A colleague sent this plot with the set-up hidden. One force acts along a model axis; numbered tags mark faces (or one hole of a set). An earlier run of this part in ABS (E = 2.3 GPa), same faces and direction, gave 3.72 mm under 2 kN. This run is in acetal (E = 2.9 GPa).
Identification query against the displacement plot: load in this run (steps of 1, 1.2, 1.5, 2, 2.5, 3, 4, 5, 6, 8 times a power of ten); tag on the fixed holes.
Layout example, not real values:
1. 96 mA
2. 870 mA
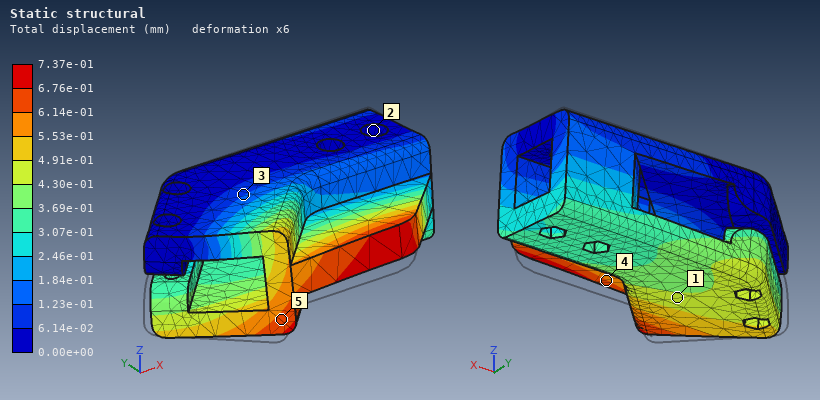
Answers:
1. 500 N
2. 2
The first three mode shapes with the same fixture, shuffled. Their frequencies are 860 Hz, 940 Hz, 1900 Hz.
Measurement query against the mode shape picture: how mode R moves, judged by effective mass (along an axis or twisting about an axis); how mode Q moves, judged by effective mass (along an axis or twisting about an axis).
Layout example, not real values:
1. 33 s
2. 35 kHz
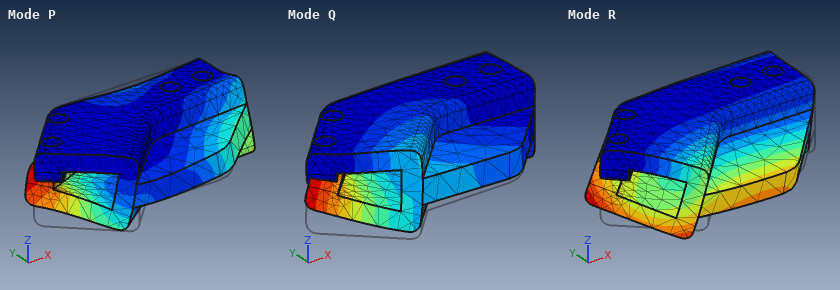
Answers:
1. along Y
2. along Z
